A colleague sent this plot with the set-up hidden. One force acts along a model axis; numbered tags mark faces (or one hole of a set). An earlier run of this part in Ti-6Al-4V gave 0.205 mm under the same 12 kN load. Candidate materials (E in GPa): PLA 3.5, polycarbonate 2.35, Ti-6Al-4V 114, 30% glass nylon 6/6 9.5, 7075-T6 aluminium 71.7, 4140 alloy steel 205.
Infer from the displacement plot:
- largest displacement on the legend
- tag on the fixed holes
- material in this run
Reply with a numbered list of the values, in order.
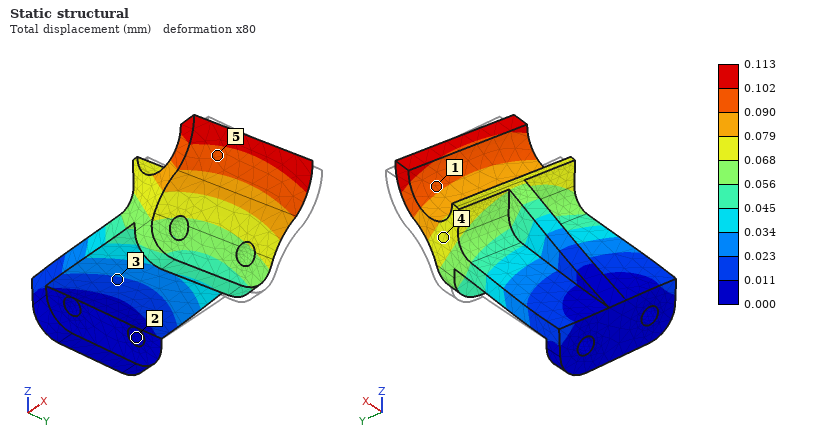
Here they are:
1. 0.113 mm
2. 2
3. 4140 alloy steel
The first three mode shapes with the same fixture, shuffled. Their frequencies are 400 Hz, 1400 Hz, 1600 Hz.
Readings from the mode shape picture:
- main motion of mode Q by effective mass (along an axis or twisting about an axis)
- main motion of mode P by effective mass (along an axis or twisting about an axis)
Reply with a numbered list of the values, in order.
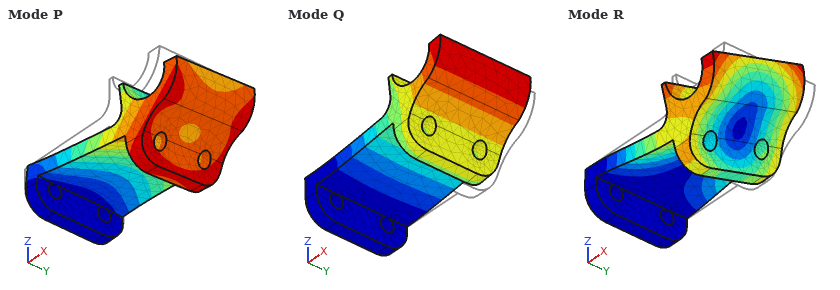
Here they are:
1. along Z
2. along Y
